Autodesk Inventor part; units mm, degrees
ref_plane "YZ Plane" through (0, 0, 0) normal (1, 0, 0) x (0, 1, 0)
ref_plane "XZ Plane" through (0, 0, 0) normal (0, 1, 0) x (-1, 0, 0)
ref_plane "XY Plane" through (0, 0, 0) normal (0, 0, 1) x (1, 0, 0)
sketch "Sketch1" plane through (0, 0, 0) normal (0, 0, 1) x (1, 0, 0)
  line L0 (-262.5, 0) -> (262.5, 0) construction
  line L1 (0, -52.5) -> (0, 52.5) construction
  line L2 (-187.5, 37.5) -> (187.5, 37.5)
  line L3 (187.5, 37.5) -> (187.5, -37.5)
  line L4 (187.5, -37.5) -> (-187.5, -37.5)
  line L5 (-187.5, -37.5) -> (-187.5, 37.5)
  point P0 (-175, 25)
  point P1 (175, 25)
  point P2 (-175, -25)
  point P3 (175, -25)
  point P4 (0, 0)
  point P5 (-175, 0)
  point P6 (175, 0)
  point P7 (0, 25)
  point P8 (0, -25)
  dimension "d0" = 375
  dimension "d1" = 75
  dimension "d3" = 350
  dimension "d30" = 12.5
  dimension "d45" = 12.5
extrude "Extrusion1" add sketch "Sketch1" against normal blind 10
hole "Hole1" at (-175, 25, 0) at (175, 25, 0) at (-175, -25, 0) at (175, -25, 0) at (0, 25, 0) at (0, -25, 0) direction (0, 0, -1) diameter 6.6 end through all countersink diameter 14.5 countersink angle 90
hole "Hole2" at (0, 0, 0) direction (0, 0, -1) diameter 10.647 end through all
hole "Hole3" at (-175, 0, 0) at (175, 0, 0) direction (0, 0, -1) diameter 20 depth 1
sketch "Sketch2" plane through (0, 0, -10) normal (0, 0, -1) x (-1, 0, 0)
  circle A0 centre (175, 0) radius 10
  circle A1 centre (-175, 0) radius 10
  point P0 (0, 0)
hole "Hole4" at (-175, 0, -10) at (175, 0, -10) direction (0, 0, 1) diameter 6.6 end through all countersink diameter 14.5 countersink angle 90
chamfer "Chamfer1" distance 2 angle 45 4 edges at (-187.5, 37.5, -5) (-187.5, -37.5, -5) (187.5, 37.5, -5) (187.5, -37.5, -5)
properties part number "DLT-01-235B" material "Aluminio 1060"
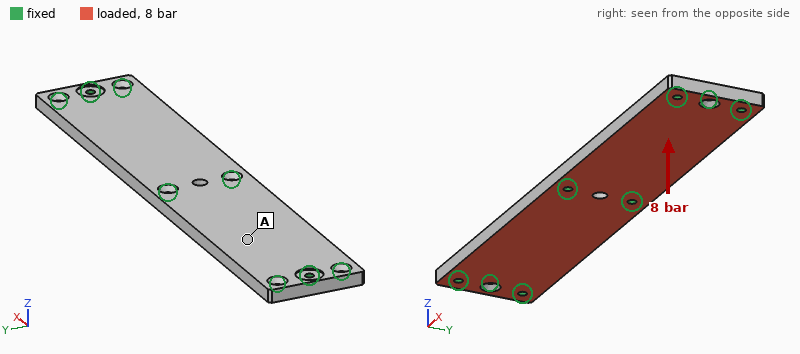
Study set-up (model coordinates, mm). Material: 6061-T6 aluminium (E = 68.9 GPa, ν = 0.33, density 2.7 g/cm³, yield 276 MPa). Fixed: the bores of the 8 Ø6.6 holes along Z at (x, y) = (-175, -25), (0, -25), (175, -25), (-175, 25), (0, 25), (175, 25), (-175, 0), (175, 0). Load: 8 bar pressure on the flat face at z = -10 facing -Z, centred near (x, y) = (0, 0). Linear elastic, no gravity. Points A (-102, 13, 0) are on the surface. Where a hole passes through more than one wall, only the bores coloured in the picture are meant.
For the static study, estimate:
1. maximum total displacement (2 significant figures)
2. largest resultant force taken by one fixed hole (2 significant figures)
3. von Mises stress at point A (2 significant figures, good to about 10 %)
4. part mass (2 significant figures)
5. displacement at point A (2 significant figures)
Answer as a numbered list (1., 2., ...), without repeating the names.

1. 0.42 mm
2. 5.4 kN
3. 60 MPa
4. 740 g
5. 0.38 mm
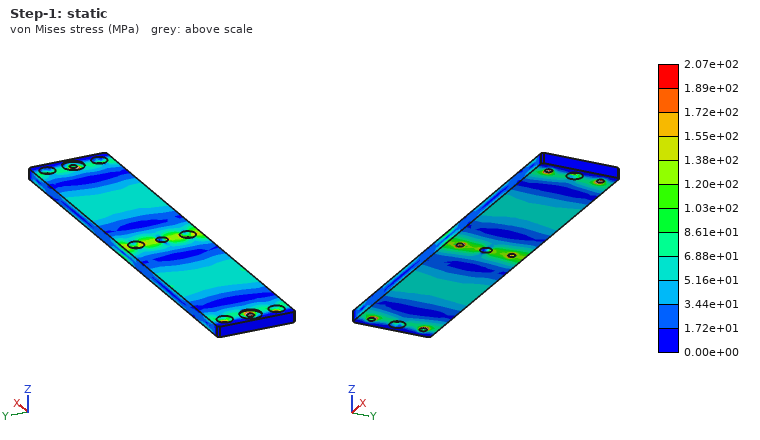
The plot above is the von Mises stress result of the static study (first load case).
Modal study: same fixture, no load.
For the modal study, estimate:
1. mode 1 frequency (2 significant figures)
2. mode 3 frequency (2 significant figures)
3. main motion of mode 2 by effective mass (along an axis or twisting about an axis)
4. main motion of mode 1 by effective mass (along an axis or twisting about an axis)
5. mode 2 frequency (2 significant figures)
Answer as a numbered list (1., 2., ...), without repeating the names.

1. 1400 Hz
2. 2700 Hz
3. along Z
4. twisting about Y
5. 1600 Hz
